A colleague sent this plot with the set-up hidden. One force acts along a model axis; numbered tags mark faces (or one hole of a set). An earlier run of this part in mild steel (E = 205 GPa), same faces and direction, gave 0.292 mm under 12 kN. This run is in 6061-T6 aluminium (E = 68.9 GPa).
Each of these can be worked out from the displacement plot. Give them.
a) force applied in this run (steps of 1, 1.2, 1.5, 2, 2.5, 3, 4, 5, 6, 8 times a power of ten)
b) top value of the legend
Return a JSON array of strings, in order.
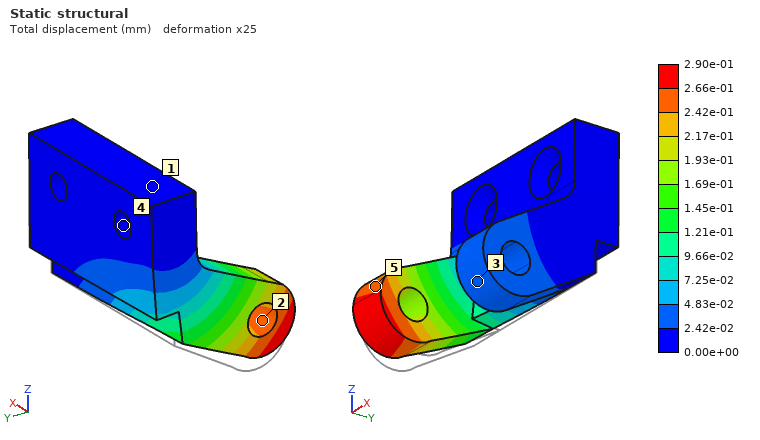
["4 kN", "2.90e-01 mm"]
